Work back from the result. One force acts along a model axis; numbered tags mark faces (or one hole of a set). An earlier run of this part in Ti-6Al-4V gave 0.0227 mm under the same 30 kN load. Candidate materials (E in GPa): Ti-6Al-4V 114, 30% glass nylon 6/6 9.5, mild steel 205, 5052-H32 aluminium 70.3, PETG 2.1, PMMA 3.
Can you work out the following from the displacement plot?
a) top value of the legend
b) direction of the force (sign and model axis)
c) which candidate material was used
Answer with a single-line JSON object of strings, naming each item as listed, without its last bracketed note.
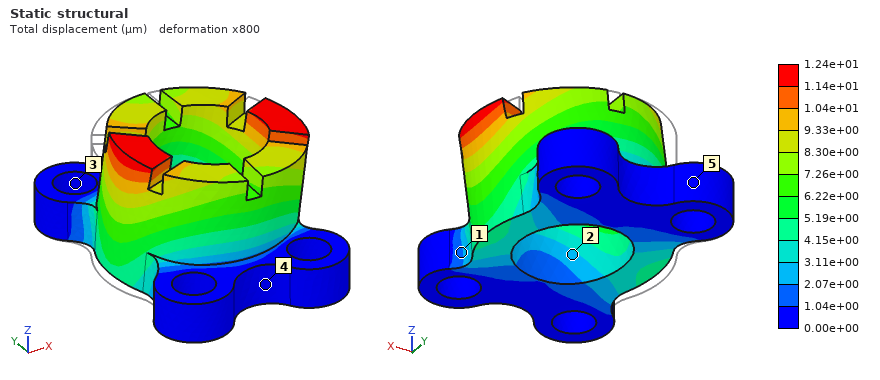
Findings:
{"top value of the legend": "1.24e+01 µm", "direction of the force": "+X", "which candidate material was used": "mild steel"}
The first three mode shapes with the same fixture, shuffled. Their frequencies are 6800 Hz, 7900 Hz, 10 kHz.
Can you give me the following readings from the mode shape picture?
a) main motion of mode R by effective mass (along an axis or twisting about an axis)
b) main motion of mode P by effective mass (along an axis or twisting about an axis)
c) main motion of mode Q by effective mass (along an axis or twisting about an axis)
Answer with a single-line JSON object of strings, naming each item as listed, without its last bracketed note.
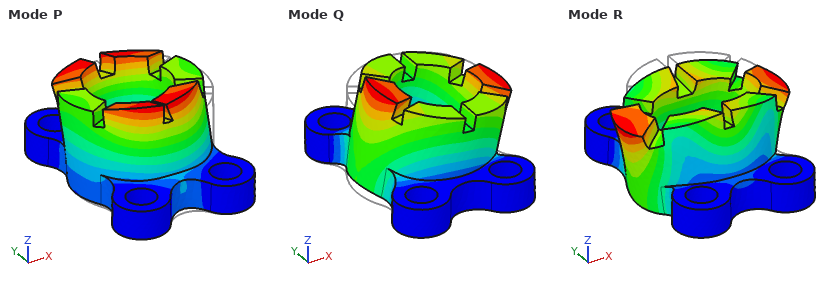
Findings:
{"main motion of mode R by effective mass": "along Z", "main motion of mode P by effective mass": "along Y", "main motion of mode Q by effective mass": "along X"}
